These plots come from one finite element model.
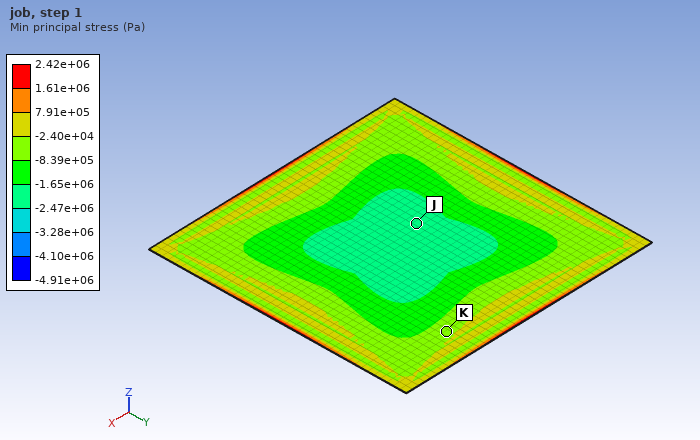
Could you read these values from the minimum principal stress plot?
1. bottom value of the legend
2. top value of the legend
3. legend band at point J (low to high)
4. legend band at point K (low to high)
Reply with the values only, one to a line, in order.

-4.91e+06 Pa
2.42e+06 Pa
-2.47e+06 to -1.65e+06 Pa
-8.39e+05 to -2.40e+04 Pa
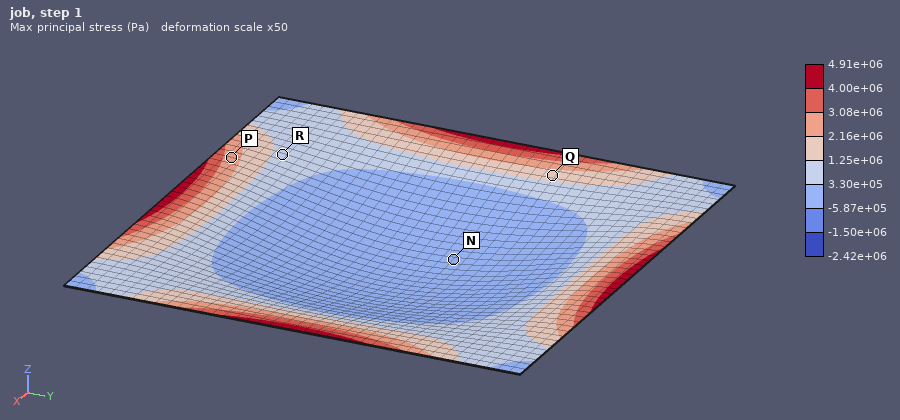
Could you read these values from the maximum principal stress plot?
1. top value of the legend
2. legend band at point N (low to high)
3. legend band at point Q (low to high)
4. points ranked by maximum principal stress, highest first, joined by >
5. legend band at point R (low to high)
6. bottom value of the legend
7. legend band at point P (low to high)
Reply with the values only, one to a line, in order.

4.91e+06 Pa
-5.87e+05 to 3.30e+05 Pa
1.25e+06 to 2.16e+06 Pa
P > Q > R > N
3.30e+05 to 1.25e+06 Pa
-2.42e+06 Pa
2.16e+06 to 3.08e+06 Pa
